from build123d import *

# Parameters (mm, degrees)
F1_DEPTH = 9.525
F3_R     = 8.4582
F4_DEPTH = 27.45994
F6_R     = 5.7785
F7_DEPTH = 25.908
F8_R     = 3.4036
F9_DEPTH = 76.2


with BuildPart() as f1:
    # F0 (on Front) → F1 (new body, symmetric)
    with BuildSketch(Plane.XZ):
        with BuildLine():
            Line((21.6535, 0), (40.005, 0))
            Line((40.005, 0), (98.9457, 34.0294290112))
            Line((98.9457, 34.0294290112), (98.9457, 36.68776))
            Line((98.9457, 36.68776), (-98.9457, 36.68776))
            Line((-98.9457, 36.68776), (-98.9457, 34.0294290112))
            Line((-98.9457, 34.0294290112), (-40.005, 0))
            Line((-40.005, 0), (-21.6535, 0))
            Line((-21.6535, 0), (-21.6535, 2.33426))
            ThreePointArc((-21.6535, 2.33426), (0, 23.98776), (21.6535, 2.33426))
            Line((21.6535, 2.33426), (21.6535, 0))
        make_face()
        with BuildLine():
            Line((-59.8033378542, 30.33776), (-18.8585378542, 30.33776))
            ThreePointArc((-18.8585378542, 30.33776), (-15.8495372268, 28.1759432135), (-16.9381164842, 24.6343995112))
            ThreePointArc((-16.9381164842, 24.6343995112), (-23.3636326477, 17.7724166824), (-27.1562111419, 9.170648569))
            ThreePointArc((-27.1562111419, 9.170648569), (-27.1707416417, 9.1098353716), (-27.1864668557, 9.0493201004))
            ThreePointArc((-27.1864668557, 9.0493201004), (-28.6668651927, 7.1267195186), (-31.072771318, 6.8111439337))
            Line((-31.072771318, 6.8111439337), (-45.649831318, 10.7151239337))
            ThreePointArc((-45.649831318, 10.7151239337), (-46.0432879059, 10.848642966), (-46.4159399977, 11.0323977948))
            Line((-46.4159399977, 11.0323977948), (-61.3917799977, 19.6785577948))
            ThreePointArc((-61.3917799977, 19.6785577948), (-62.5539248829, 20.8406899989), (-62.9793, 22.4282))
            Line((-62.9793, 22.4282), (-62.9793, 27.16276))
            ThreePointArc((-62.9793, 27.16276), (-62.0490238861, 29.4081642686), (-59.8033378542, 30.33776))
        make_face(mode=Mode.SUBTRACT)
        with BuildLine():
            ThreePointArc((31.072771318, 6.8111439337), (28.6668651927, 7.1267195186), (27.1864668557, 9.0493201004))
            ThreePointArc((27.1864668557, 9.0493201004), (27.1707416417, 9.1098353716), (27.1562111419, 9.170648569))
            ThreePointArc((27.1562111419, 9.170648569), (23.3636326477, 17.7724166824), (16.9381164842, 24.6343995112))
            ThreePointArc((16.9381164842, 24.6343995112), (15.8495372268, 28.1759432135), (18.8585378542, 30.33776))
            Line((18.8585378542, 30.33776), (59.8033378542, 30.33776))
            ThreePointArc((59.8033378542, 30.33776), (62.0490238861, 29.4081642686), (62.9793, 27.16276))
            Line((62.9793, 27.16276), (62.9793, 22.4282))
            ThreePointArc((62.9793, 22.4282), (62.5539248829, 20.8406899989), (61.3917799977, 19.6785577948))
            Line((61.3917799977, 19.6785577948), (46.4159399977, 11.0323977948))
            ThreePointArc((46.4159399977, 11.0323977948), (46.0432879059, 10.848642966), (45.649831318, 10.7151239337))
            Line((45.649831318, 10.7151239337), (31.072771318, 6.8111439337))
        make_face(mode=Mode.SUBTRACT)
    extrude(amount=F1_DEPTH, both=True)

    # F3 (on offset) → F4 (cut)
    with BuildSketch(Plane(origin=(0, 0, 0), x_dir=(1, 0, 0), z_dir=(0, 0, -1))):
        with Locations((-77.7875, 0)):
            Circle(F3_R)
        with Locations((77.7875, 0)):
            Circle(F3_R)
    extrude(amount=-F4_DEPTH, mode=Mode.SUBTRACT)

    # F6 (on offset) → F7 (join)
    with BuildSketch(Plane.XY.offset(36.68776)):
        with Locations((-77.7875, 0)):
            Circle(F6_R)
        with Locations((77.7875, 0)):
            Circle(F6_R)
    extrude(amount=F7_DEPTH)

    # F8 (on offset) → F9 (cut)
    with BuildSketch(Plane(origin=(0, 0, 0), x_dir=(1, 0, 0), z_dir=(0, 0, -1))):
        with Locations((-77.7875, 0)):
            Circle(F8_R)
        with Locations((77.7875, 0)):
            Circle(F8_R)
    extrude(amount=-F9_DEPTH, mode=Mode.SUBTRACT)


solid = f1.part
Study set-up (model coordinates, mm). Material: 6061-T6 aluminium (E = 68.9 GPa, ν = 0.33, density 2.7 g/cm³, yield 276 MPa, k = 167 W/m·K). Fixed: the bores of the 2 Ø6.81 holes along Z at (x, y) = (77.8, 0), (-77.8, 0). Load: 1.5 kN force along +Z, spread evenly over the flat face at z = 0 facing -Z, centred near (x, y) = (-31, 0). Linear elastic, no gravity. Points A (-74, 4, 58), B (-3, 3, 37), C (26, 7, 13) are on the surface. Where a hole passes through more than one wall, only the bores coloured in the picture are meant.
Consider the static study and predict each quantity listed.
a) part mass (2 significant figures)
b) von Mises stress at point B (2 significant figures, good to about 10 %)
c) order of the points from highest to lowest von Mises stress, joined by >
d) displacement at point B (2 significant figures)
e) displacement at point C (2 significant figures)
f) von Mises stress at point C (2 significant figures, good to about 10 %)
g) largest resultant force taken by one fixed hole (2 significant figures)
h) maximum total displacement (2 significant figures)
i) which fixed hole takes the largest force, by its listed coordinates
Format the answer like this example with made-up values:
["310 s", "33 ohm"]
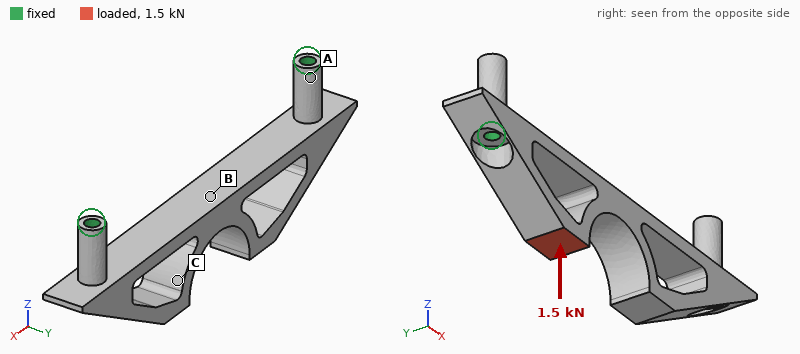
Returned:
["150 g", "30 MPa", "B > C > A", "0.19 mm", "0.15 mm", "19 MPa", "1.1 kN", "0.20 mm", "(-77.8, 0)"]
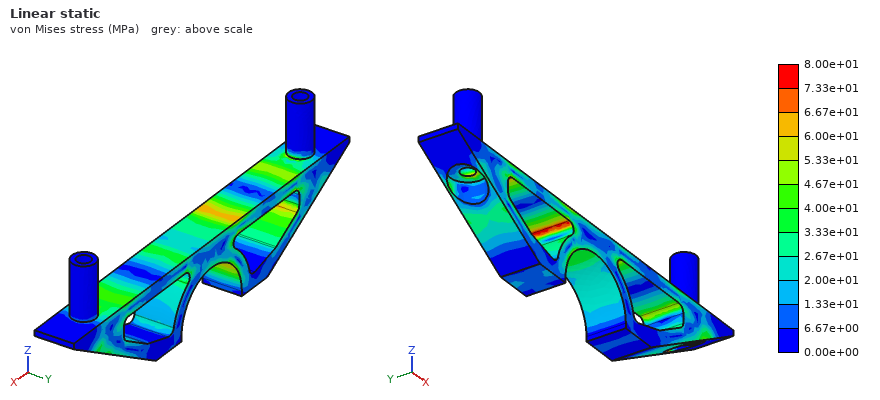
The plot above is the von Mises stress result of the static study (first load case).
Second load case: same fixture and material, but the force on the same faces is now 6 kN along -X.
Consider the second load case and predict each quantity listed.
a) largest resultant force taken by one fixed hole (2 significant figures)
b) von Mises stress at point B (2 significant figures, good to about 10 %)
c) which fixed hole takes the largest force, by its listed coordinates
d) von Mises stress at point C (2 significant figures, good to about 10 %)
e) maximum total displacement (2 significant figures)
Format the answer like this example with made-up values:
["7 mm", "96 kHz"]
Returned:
["4.6 kN", "77 MPa", "(-77.8, 0)", "48 MPa", "0.47 mm"]
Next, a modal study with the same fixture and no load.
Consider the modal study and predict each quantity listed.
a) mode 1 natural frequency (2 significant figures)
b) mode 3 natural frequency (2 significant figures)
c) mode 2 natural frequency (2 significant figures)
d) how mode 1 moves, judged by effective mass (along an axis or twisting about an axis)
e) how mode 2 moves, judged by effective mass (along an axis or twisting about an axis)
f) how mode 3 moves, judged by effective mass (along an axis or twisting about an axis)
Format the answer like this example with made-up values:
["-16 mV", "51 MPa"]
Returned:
["1600 Hz", "4400 Hz", "2600 Hz", "along Z", "along Y", "twisting about X"]
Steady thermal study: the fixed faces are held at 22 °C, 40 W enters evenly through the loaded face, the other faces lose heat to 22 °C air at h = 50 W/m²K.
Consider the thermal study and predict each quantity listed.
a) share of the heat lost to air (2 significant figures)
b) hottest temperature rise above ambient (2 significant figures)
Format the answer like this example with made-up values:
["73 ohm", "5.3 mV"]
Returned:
["27 %", "45 K"]
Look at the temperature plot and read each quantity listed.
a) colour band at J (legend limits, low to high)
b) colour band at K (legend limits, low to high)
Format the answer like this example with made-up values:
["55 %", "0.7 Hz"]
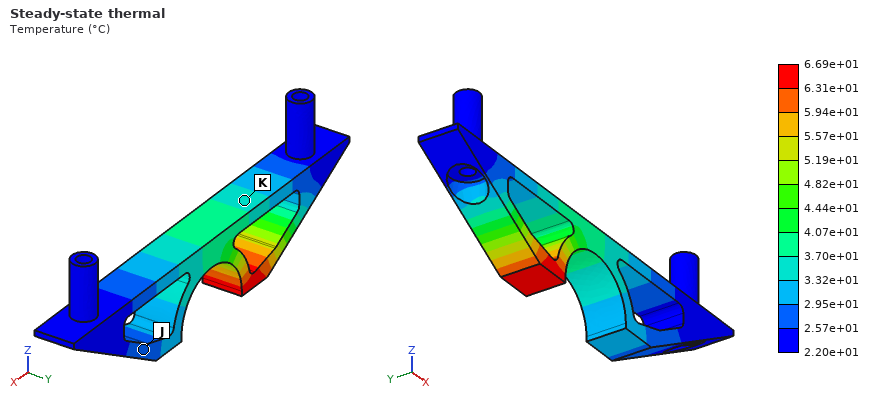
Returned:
["2.57e+01 to 2.95e+01 °C", "3.32e+01 to 3.70e+01 °C"]
